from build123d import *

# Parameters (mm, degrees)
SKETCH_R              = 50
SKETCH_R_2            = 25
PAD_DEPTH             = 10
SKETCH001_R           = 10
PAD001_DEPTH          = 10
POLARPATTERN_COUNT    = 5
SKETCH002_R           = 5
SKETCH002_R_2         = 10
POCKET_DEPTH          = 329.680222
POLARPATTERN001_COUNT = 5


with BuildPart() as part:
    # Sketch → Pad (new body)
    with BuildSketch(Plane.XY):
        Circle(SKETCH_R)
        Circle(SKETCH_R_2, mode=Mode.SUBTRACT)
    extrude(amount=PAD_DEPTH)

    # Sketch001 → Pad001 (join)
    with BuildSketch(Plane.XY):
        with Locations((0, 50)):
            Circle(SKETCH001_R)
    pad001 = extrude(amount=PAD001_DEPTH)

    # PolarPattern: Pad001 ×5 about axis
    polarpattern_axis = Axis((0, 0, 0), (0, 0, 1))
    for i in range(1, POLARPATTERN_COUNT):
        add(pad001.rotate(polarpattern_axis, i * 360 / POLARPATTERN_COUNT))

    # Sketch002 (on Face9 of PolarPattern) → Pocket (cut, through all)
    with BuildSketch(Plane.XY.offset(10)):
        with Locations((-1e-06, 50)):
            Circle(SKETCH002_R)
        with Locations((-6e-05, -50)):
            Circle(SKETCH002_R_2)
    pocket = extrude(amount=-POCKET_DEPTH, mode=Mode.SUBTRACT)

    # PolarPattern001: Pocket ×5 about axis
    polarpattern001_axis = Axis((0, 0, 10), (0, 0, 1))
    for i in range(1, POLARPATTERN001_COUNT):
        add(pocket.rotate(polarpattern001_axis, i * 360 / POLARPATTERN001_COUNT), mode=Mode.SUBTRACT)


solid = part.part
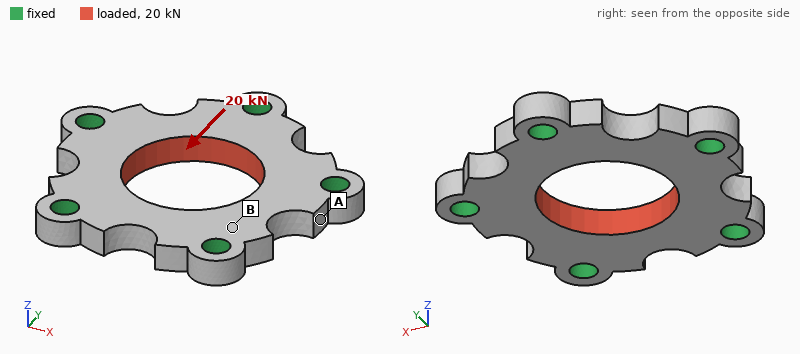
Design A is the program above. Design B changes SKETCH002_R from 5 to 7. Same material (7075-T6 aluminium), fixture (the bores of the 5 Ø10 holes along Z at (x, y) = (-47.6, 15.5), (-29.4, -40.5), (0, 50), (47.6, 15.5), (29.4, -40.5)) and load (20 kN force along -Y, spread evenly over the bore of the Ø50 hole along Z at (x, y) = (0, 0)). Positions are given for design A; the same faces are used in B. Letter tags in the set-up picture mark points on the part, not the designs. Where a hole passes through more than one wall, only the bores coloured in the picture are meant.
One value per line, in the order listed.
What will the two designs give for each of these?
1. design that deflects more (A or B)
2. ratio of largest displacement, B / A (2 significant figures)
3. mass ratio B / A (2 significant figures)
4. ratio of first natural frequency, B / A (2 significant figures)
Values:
A
0.87
0.93
1.2
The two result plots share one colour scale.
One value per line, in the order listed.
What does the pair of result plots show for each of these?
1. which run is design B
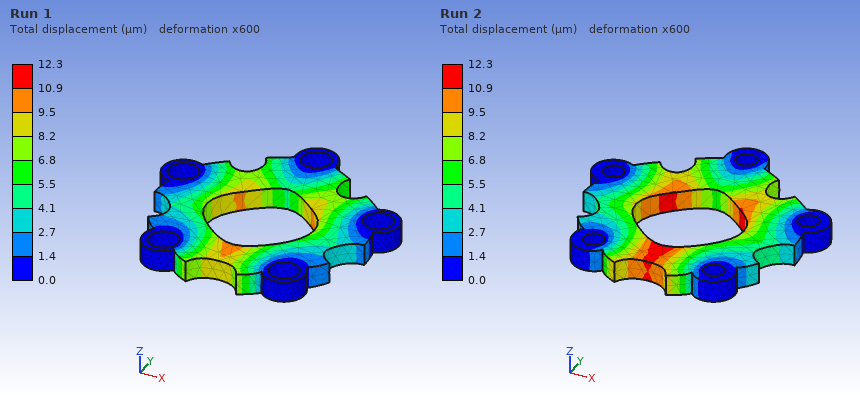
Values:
Run 1
